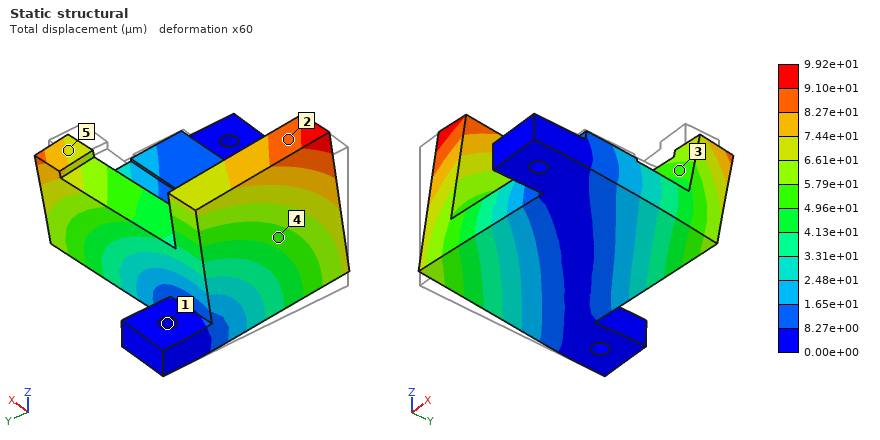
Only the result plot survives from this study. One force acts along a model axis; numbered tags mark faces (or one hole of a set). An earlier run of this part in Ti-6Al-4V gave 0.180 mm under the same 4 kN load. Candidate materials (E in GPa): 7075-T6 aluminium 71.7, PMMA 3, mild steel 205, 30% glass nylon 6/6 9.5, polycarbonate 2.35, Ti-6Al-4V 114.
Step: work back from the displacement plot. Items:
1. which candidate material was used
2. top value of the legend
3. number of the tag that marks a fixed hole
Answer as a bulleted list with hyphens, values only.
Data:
- mild steel
- 9.92e+01 µm
- 1
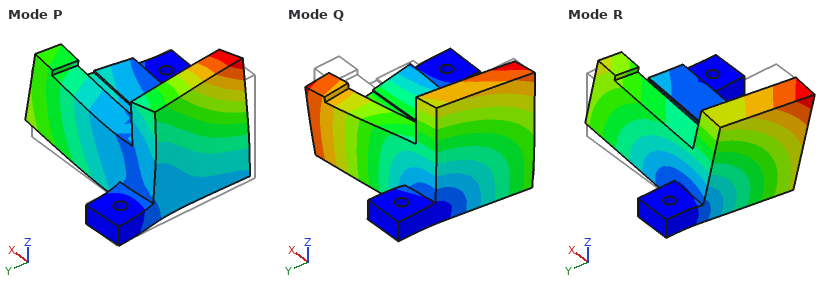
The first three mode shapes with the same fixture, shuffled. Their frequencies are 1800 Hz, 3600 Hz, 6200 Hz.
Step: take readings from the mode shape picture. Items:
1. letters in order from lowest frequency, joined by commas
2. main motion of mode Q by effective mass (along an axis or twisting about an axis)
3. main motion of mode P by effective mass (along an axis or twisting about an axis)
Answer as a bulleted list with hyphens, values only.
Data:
- R, Q, P
- along Z
- along X
